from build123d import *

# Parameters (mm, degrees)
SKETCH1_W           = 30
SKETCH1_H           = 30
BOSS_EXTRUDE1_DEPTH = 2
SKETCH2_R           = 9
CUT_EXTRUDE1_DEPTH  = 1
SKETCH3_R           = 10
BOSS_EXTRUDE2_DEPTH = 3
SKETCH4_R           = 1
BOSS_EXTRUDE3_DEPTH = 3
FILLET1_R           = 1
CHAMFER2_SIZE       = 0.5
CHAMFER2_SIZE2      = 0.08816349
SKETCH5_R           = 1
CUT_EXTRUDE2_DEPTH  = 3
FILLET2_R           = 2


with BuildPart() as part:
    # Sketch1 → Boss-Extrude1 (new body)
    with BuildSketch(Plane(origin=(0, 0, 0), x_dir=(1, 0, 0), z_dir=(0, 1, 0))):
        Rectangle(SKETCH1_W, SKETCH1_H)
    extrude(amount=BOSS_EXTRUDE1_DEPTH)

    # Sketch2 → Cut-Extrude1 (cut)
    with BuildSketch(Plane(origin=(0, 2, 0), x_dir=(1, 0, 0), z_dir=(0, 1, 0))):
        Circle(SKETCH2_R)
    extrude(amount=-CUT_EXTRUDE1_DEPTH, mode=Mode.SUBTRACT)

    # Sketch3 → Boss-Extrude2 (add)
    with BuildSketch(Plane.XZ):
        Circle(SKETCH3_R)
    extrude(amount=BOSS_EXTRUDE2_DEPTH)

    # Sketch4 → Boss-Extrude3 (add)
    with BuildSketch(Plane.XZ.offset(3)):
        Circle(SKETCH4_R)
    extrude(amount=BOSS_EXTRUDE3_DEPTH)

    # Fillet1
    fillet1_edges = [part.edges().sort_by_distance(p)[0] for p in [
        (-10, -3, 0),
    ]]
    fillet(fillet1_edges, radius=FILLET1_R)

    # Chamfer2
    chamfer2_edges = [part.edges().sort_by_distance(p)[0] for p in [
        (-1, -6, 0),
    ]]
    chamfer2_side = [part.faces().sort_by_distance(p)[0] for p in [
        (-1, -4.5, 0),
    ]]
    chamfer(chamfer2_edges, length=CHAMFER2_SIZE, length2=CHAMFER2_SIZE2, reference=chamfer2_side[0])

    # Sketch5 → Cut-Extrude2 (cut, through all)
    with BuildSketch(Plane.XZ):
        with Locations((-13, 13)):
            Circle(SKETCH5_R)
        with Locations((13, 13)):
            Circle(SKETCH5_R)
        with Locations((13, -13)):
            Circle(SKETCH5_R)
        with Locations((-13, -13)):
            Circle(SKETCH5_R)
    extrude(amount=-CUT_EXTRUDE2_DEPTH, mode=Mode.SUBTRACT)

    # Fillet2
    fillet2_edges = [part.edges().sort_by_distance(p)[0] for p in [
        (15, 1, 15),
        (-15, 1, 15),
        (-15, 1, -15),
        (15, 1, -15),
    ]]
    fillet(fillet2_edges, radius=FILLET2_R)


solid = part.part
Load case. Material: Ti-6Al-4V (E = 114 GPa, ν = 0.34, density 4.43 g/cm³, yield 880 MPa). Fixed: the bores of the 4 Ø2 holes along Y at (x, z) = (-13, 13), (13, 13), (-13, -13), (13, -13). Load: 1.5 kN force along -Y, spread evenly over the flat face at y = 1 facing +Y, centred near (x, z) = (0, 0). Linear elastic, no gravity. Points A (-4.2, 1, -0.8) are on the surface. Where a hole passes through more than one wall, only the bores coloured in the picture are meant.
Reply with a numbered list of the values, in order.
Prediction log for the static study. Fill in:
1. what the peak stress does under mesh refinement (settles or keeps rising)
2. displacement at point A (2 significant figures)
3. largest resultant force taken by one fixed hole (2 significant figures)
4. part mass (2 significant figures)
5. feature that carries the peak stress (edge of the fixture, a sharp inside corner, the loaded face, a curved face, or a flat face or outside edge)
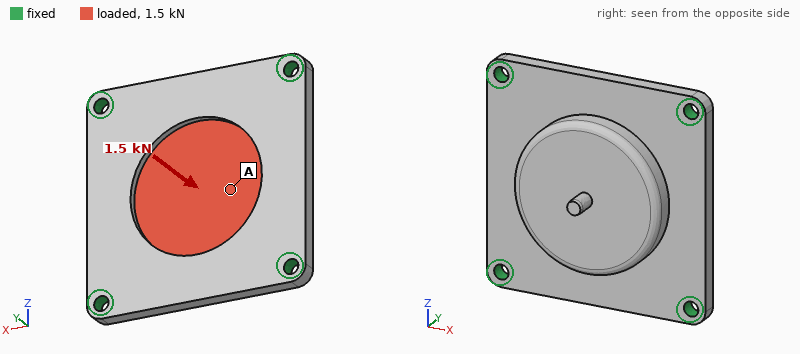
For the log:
1. keeps rising
2. 49 µm
3. 510 N
4. 11 g
5. edge of the fixture
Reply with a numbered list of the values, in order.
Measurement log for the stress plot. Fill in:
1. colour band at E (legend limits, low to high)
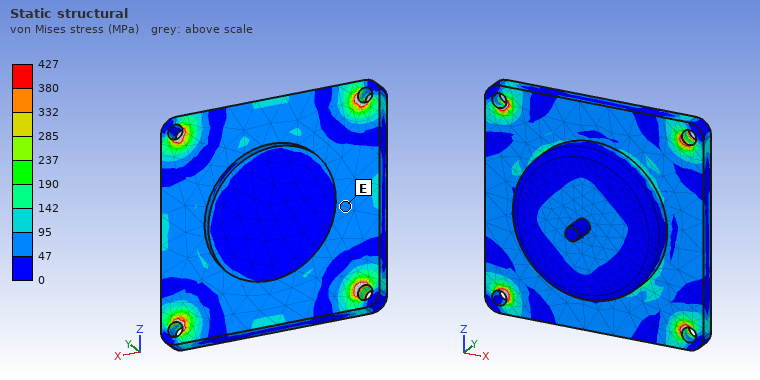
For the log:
1. 47 to 95 MPa
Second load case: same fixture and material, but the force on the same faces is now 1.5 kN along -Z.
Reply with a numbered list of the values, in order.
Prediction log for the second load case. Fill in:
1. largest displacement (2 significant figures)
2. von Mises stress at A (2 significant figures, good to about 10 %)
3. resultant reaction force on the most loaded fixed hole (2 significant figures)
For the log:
1. 5.0 µm
2. 18 MPa
3. 410 N
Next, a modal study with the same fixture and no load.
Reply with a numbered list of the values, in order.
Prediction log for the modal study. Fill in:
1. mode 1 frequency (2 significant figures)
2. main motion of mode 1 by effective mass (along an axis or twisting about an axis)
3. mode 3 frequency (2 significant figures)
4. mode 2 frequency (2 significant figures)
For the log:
1. 10 kHz
2. along Y
3. 16 kHz
4. 16 kHz
